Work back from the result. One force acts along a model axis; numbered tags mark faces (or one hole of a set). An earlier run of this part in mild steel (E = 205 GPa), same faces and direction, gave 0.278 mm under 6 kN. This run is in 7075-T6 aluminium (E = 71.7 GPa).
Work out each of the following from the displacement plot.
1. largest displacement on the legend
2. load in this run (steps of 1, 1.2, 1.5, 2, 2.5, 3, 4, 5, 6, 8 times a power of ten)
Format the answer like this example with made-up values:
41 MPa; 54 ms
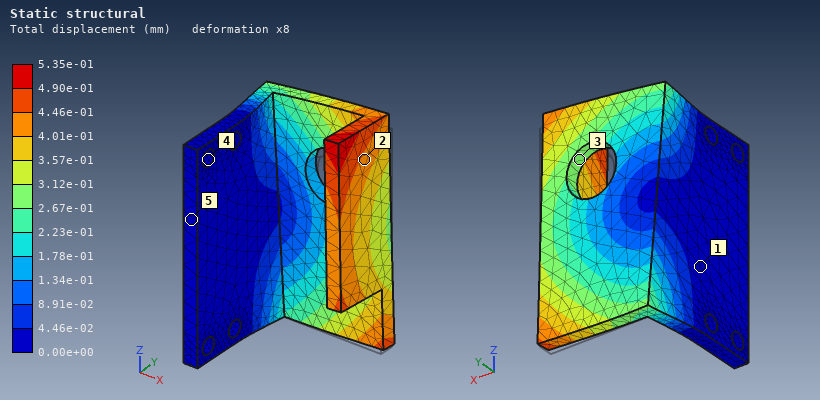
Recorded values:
5.35e-01 mm; 4 kN
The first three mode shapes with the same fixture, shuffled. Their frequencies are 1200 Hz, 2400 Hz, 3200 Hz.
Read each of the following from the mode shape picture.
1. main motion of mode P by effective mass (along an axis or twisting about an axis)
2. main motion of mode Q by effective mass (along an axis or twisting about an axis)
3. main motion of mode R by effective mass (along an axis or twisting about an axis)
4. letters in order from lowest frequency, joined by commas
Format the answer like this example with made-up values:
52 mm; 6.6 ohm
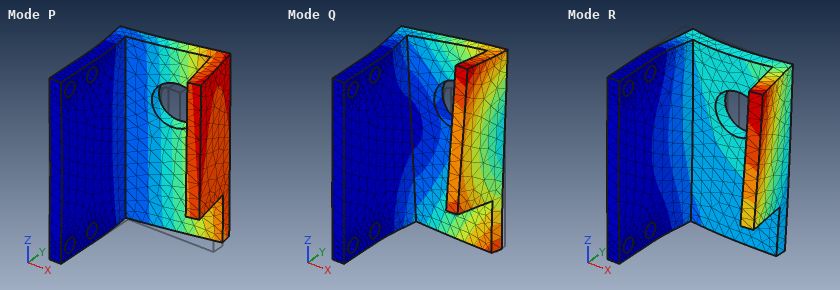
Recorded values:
along Y; along Z; along X; P, Q, R
